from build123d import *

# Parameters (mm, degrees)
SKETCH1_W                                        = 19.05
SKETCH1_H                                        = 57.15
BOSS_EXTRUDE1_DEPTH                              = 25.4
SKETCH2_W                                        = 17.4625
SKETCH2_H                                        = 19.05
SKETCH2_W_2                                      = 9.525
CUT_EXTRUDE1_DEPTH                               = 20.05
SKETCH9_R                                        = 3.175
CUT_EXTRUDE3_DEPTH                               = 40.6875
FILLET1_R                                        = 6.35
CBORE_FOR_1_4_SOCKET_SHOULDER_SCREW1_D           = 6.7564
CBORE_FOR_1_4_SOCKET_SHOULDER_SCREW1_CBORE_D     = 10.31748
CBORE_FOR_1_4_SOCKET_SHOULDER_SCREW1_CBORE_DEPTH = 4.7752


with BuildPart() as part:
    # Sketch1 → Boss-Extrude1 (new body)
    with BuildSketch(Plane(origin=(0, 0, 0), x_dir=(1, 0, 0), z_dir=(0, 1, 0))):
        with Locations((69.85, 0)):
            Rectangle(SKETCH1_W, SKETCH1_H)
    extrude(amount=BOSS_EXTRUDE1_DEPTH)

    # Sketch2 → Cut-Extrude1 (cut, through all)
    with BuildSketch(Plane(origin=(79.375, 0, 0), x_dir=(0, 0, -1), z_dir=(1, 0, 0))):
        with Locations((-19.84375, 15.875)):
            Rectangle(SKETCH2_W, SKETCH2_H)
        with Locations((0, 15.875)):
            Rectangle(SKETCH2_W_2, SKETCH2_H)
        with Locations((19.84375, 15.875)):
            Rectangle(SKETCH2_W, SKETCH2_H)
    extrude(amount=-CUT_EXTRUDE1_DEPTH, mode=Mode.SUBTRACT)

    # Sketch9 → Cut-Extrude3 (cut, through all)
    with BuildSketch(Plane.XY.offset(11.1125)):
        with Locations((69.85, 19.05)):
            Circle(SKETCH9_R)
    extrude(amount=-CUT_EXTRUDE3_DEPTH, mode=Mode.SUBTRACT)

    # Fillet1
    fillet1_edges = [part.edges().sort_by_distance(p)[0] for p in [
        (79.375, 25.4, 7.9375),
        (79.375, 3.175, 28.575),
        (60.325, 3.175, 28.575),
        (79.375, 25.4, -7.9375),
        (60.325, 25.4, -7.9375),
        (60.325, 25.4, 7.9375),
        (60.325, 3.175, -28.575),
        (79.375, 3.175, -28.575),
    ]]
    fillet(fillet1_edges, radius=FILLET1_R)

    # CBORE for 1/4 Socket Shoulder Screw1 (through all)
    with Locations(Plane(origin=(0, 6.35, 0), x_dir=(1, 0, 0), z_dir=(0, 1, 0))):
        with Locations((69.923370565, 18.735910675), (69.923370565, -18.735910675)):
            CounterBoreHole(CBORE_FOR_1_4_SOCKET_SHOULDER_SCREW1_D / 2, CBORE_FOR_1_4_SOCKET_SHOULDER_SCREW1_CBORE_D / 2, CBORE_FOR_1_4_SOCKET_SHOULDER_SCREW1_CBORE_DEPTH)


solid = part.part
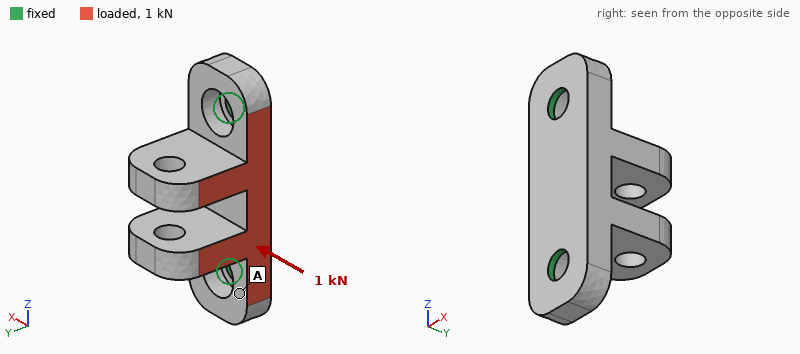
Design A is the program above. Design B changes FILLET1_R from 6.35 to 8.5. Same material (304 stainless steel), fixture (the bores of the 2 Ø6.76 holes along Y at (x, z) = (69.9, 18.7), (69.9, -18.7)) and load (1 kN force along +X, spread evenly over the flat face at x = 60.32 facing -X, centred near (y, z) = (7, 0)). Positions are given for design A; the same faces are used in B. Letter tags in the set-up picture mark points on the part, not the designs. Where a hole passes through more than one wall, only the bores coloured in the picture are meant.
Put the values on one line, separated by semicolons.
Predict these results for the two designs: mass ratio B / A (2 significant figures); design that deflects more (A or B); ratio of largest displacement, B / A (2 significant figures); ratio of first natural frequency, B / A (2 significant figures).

0.96; A; 0.91; 1.0
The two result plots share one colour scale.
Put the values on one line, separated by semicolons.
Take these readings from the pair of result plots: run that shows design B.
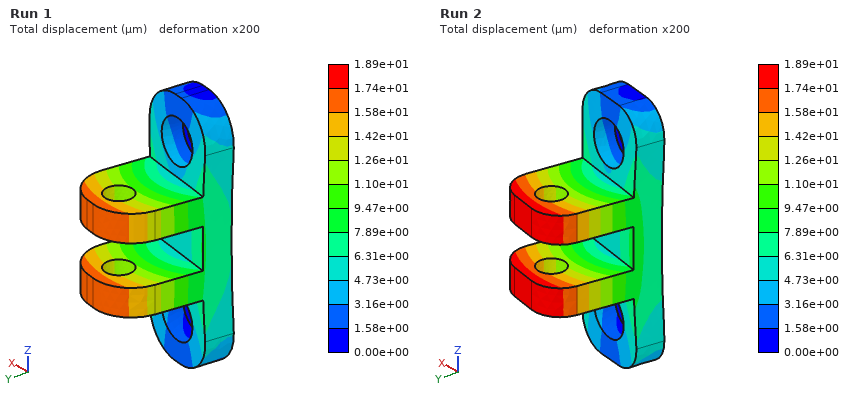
Run 1
